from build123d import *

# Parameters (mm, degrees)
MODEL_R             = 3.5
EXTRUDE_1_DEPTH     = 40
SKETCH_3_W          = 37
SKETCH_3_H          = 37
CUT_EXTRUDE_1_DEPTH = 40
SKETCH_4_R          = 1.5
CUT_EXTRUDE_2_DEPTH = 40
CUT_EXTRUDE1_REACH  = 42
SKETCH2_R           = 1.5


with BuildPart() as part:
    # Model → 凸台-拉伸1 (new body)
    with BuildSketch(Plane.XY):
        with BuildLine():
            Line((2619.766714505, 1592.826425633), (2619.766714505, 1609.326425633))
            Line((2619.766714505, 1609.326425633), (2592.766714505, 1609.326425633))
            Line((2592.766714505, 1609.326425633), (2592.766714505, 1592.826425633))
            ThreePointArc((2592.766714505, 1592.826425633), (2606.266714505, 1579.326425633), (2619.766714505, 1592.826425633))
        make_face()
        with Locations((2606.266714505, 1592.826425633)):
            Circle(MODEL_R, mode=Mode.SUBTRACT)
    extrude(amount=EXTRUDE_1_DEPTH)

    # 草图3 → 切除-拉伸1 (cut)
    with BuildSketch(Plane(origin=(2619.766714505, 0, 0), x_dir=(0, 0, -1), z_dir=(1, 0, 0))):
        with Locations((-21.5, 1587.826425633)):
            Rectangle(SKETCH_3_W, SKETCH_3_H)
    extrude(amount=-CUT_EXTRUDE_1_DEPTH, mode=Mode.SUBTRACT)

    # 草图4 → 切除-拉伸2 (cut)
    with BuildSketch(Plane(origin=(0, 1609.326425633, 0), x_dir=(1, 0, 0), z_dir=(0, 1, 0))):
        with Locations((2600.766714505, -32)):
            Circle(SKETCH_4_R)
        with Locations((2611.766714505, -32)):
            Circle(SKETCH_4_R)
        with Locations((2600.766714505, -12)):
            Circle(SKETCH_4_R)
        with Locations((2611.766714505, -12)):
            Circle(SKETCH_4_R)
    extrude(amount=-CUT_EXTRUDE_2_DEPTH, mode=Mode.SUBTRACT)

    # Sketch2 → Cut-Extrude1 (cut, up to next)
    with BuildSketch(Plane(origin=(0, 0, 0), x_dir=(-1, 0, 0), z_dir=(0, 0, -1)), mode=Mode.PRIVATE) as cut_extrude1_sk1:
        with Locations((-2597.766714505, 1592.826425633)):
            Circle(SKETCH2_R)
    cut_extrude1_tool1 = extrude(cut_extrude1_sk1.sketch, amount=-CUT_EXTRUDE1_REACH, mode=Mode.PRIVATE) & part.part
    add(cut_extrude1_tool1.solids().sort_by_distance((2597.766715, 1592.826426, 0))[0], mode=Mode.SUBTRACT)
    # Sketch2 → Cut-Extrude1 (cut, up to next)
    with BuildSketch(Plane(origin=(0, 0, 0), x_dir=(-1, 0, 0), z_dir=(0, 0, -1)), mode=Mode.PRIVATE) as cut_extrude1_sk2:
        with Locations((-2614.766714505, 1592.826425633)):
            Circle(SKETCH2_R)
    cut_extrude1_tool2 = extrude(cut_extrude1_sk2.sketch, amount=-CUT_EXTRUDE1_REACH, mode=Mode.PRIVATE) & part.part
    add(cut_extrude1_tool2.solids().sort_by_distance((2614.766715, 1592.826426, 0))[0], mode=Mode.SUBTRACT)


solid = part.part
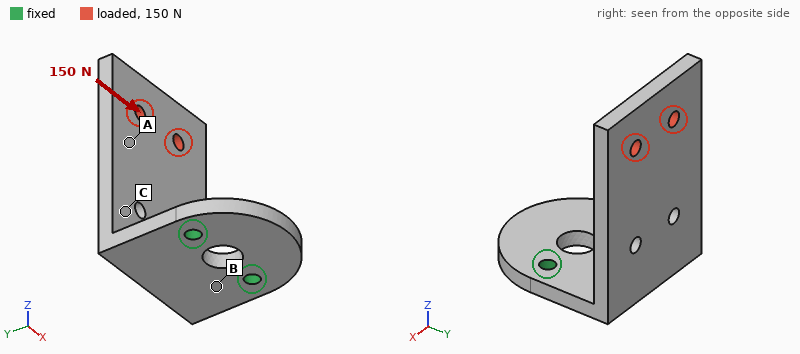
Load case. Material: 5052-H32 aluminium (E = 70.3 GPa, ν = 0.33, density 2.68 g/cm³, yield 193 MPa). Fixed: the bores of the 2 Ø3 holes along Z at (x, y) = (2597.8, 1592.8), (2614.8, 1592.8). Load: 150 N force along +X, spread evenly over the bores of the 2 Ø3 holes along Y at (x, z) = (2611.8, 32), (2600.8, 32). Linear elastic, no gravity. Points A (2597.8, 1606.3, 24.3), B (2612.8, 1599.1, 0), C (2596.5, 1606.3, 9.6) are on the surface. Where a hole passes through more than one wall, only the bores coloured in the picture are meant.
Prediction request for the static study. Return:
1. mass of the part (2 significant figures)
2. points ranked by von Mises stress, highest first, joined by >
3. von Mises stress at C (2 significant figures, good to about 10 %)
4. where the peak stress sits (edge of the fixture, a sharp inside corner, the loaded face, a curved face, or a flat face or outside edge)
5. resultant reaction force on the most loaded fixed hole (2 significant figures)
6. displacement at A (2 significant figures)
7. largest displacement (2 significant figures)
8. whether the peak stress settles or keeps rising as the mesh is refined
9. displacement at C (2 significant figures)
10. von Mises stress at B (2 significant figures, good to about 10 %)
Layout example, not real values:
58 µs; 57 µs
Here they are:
13 g; B > C > A; 27 MPa; edge of the fixture; 260 N; 0.13 mm; 0.21 mm; keeps rising; 0.064 mm; 49 MPa
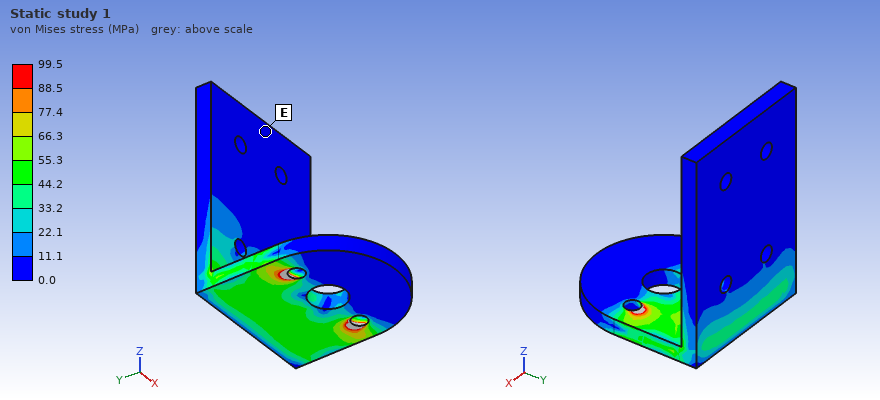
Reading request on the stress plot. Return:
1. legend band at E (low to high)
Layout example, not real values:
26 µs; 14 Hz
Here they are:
0.0 to 11.1 MPa
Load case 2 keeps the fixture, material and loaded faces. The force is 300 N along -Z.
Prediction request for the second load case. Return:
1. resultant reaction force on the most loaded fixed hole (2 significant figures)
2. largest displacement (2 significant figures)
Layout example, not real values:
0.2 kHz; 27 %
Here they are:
150 N; 0.33 mm
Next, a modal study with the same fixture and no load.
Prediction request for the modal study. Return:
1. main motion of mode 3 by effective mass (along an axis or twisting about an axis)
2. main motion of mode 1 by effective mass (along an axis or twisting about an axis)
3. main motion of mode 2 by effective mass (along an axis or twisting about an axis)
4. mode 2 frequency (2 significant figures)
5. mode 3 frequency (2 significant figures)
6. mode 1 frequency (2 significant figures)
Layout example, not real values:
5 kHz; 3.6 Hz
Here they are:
along Z; along Y; along X; 2200 Hz; 4200 Hz; 1000 Hz
